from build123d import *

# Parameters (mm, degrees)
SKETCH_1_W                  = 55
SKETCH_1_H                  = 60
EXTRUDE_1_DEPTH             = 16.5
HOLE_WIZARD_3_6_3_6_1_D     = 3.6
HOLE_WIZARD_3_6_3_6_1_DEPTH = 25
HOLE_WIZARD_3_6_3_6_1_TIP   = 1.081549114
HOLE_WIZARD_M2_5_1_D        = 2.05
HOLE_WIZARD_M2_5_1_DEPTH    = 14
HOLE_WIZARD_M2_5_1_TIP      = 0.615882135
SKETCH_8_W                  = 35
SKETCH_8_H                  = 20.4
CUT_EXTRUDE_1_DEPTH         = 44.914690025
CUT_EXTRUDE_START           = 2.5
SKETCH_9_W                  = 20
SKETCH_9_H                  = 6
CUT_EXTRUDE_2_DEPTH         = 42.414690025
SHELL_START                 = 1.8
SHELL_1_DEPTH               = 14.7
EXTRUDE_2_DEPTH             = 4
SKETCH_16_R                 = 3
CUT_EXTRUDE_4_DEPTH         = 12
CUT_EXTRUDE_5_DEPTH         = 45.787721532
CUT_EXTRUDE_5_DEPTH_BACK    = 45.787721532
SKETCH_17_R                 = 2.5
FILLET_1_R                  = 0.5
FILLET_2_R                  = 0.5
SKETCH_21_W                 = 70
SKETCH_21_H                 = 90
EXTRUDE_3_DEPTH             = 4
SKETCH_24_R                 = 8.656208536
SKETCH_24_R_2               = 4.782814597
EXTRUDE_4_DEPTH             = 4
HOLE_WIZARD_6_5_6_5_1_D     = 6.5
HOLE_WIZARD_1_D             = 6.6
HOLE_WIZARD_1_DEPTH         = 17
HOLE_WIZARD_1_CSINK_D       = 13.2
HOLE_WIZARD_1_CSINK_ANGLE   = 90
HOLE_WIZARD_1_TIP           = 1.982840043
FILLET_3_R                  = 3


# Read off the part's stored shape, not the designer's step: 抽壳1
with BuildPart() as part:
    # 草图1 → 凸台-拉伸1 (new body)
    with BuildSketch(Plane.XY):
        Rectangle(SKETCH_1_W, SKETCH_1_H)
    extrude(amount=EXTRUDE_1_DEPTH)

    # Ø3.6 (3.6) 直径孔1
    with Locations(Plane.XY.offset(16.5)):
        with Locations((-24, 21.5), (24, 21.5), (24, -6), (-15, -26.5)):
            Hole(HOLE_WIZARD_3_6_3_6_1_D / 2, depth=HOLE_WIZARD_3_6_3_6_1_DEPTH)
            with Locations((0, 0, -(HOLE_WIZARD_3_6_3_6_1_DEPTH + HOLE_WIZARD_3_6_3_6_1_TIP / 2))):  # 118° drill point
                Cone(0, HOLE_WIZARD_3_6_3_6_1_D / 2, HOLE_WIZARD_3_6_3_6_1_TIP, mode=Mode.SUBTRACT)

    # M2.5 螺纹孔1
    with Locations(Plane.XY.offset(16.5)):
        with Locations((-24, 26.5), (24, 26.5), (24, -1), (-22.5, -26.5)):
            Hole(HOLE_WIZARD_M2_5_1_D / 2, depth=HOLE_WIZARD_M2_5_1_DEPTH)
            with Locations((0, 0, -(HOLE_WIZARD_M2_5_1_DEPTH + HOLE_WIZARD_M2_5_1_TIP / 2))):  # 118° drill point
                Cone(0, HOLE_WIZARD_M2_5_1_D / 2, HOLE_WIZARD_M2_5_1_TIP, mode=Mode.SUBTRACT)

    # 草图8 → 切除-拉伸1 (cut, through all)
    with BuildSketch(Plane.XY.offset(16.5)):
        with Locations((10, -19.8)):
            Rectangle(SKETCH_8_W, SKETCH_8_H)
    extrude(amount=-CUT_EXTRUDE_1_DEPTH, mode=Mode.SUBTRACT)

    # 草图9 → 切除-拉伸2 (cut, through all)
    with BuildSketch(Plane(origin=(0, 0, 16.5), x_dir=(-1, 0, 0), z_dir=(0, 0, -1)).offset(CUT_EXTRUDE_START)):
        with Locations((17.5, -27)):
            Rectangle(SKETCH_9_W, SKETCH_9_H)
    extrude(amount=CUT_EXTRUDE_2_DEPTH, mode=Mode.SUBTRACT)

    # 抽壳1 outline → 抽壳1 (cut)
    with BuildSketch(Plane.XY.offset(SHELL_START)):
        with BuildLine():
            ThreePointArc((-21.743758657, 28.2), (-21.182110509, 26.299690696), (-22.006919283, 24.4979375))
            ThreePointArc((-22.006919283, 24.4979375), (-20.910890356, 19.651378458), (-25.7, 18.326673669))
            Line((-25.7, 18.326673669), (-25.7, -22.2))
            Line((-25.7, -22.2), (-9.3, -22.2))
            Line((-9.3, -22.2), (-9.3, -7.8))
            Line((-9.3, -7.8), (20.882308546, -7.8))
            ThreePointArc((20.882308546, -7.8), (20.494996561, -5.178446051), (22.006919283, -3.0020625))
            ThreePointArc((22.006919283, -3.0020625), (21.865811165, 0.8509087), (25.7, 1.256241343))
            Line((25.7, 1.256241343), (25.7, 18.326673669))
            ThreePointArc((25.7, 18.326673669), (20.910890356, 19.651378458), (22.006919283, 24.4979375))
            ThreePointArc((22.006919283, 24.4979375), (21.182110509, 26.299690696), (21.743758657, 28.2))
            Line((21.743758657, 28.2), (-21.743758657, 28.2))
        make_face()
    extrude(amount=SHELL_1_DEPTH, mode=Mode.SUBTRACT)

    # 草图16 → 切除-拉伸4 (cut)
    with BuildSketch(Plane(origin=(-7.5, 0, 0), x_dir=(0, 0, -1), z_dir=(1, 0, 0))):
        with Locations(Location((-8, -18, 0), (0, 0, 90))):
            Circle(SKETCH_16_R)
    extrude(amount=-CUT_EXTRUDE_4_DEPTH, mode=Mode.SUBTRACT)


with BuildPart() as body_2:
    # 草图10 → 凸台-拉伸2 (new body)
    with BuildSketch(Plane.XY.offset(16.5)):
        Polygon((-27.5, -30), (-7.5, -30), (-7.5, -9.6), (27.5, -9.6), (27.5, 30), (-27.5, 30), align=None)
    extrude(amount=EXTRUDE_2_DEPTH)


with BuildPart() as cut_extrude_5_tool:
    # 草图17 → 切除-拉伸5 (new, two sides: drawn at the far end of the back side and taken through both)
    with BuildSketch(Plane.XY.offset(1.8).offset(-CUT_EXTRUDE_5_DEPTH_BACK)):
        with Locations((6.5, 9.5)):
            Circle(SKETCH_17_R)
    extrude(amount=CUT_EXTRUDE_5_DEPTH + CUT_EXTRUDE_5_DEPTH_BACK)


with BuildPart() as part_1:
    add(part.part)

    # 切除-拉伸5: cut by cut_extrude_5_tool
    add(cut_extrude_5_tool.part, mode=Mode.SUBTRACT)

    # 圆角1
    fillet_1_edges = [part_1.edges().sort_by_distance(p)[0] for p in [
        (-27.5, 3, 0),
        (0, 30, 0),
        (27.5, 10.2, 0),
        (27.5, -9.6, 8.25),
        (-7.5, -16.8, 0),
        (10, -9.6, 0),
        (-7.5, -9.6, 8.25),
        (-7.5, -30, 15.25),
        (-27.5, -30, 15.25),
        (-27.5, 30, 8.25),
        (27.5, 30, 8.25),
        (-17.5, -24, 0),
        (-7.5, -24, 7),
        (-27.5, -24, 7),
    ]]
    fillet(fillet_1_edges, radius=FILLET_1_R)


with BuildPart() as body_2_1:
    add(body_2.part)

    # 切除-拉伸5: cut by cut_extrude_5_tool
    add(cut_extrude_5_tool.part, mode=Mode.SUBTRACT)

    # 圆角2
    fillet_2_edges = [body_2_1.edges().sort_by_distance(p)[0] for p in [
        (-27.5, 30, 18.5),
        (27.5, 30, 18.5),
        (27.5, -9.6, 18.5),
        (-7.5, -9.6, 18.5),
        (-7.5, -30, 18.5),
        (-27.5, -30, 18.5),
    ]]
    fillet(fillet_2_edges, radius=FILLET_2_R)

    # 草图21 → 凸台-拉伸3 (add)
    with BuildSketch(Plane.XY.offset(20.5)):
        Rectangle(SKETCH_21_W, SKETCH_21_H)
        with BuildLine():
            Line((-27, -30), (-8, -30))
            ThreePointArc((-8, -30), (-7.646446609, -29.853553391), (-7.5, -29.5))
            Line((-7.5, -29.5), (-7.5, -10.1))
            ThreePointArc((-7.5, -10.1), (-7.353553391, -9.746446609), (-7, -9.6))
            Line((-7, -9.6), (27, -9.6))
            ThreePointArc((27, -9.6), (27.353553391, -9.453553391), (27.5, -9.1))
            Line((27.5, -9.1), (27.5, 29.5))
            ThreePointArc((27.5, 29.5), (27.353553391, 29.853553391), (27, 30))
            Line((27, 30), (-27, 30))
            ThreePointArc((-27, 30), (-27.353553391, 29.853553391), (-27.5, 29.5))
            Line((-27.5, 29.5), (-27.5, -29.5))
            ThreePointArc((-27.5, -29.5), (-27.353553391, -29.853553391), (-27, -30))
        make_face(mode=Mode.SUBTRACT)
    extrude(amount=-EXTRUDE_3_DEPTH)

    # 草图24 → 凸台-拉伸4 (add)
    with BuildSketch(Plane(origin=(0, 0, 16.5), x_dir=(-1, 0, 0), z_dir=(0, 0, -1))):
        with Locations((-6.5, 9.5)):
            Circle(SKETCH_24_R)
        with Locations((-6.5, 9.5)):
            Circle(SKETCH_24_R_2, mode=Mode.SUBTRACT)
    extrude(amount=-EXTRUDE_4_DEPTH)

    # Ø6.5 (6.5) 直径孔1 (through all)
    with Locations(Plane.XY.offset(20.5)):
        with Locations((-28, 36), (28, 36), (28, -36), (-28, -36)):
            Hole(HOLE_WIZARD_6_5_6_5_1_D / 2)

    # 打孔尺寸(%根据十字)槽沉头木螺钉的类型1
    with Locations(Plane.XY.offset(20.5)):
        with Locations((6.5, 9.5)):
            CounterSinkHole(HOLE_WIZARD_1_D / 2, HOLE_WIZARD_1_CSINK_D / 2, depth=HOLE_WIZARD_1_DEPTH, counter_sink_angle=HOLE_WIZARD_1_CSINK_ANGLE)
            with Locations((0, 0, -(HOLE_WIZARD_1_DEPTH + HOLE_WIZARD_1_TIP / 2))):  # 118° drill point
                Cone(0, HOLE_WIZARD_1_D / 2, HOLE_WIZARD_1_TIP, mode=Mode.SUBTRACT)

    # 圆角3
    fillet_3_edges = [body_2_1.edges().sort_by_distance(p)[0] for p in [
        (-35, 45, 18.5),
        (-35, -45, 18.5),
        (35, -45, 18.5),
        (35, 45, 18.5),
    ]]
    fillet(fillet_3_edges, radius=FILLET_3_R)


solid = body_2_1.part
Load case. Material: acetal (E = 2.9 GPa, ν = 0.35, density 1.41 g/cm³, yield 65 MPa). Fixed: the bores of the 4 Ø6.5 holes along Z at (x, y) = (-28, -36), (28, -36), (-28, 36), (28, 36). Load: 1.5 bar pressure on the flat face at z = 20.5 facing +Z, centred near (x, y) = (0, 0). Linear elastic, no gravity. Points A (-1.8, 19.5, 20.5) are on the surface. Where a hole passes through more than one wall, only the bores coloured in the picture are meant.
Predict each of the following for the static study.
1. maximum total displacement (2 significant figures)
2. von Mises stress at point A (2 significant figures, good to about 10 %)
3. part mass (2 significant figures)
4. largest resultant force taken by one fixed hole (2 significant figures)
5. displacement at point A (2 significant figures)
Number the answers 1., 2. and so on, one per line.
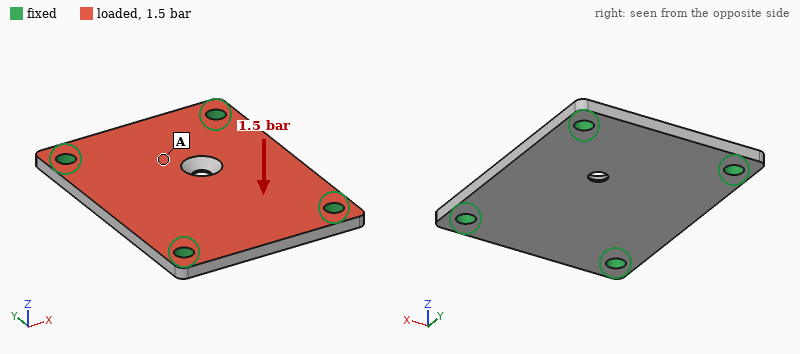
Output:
1. 0.96 mm
2. 7.7 MPa
3. 34 g
4. 230 N
5. 0.67 mm
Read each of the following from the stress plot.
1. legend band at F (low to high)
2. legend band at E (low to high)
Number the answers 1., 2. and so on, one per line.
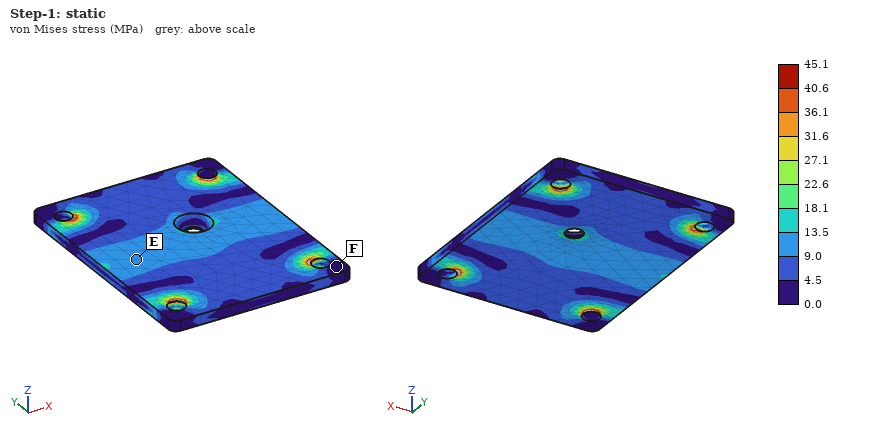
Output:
1. 0.0 to 4.5 MPa
2. 9.0 to 13.5 MPa
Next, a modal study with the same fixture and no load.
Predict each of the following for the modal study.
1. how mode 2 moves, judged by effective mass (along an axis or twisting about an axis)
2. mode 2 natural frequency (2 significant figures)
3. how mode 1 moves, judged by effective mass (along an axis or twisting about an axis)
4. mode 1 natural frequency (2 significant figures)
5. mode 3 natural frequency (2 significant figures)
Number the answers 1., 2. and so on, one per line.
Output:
1. twisting about Y
2. 1500 Hz
3. along Z
4. 1000 Hz
5. 1900 Hz
